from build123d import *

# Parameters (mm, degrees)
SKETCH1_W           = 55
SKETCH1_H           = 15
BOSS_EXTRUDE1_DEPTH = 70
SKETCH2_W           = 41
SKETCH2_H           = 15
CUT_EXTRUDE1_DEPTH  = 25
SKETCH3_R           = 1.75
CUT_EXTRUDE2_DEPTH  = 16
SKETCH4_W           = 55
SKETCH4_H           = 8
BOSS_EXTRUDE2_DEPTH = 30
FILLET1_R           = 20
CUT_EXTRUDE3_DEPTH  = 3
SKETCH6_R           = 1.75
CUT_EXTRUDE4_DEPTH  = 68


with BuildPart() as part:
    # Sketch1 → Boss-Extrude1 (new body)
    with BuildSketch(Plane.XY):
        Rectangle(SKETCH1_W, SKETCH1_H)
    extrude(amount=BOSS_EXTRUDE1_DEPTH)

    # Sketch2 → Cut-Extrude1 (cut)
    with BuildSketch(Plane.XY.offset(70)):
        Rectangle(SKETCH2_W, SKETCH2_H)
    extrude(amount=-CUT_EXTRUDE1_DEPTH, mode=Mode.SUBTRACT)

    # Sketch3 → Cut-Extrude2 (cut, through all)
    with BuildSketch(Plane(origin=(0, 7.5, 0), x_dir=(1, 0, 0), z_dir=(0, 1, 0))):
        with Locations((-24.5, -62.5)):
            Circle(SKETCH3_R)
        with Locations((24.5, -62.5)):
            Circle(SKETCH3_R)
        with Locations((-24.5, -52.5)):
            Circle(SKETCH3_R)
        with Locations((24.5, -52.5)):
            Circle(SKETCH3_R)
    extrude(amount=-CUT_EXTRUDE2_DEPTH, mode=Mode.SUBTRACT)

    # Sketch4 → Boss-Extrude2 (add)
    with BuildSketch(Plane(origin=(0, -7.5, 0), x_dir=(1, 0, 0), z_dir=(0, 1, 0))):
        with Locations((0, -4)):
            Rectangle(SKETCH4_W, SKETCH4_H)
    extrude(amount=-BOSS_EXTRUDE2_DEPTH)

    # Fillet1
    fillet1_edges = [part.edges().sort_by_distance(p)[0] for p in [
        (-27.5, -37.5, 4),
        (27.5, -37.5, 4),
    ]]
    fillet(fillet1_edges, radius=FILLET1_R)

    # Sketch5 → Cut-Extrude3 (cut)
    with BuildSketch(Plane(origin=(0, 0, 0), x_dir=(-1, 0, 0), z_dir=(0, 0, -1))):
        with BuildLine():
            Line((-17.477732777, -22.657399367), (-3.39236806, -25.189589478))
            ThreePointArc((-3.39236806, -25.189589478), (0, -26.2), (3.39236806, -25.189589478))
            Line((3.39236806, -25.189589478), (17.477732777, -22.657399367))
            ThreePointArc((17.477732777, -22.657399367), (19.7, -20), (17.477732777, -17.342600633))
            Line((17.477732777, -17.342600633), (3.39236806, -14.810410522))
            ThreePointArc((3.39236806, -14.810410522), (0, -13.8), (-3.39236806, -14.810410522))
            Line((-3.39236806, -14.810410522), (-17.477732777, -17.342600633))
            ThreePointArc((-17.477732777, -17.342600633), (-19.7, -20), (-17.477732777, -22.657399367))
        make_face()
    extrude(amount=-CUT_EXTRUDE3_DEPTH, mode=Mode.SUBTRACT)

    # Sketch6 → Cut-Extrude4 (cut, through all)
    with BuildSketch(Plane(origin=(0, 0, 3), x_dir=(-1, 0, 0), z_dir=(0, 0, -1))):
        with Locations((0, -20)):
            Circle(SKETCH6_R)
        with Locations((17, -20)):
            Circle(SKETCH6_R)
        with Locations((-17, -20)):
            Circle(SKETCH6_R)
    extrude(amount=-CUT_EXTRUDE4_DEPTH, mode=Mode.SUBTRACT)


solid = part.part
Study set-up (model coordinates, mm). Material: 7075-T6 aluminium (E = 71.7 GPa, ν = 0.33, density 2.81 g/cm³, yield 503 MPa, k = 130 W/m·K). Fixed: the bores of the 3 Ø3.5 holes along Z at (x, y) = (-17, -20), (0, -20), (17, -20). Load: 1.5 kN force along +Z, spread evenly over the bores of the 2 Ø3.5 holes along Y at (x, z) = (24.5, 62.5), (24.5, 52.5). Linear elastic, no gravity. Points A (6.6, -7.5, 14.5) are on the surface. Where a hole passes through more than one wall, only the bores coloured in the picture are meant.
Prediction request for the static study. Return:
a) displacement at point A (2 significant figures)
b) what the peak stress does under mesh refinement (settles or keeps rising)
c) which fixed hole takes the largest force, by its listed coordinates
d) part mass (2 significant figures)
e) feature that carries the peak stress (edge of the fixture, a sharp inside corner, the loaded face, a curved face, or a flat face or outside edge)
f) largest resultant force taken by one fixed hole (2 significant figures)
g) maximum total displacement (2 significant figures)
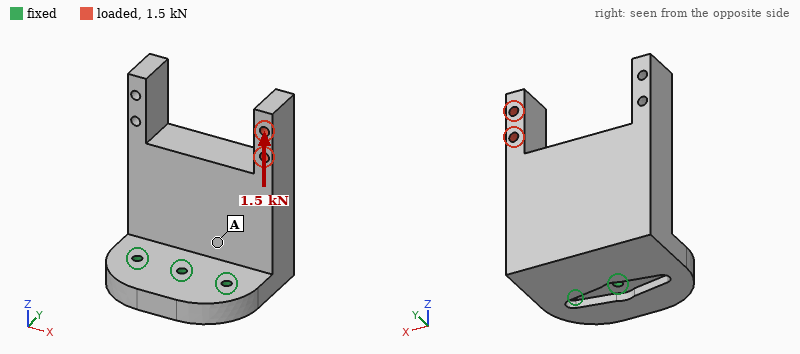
0.058 mm
keeps rising
(17, -20)
150 g
edge of the fixture
1.5 kN
0.31 mm
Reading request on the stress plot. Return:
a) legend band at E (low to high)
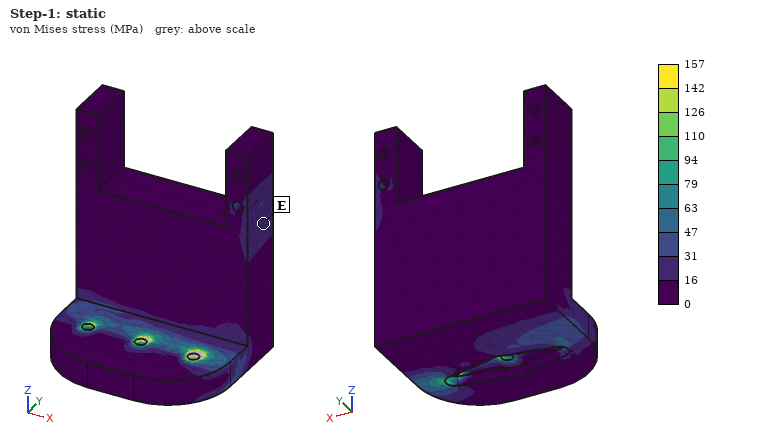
16 to 31 MPa
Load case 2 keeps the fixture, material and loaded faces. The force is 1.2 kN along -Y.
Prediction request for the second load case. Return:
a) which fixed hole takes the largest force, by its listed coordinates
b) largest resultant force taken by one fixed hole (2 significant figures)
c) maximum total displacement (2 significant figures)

(0, -20)
1.2 kN
0.93 mm
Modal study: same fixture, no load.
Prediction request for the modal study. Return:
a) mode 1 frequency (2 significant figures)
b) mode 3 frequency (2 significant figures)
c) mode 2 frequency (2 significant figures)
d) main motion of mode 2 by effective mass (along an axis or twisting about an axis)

1100 Hz
5400 Hz
2700 Hz
along X
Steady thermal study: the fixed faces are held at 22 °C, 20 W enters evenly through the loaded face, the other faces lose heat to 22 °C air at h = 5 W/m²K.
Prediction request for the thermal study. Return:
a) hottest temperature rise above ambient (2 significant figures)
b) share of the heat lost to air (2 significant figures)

49 K
3.7 %
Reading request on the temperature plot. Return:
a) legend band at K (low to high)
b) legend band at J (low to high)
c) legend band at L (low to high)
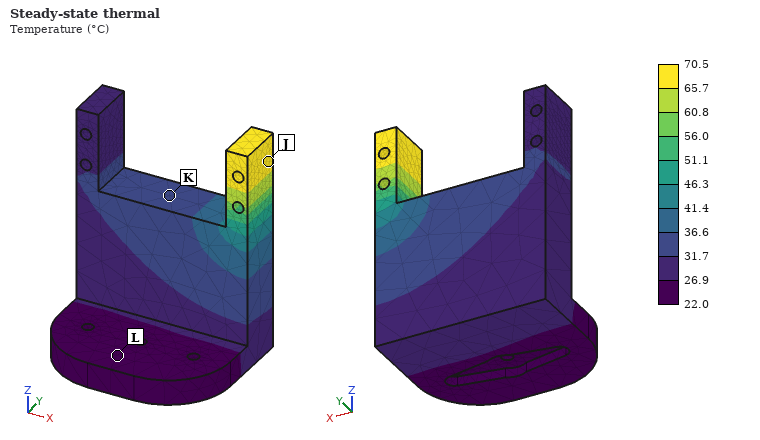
31.7 to 36.6 °C
65.7 to 70.5 °C
22.0 to 26.9 °C
